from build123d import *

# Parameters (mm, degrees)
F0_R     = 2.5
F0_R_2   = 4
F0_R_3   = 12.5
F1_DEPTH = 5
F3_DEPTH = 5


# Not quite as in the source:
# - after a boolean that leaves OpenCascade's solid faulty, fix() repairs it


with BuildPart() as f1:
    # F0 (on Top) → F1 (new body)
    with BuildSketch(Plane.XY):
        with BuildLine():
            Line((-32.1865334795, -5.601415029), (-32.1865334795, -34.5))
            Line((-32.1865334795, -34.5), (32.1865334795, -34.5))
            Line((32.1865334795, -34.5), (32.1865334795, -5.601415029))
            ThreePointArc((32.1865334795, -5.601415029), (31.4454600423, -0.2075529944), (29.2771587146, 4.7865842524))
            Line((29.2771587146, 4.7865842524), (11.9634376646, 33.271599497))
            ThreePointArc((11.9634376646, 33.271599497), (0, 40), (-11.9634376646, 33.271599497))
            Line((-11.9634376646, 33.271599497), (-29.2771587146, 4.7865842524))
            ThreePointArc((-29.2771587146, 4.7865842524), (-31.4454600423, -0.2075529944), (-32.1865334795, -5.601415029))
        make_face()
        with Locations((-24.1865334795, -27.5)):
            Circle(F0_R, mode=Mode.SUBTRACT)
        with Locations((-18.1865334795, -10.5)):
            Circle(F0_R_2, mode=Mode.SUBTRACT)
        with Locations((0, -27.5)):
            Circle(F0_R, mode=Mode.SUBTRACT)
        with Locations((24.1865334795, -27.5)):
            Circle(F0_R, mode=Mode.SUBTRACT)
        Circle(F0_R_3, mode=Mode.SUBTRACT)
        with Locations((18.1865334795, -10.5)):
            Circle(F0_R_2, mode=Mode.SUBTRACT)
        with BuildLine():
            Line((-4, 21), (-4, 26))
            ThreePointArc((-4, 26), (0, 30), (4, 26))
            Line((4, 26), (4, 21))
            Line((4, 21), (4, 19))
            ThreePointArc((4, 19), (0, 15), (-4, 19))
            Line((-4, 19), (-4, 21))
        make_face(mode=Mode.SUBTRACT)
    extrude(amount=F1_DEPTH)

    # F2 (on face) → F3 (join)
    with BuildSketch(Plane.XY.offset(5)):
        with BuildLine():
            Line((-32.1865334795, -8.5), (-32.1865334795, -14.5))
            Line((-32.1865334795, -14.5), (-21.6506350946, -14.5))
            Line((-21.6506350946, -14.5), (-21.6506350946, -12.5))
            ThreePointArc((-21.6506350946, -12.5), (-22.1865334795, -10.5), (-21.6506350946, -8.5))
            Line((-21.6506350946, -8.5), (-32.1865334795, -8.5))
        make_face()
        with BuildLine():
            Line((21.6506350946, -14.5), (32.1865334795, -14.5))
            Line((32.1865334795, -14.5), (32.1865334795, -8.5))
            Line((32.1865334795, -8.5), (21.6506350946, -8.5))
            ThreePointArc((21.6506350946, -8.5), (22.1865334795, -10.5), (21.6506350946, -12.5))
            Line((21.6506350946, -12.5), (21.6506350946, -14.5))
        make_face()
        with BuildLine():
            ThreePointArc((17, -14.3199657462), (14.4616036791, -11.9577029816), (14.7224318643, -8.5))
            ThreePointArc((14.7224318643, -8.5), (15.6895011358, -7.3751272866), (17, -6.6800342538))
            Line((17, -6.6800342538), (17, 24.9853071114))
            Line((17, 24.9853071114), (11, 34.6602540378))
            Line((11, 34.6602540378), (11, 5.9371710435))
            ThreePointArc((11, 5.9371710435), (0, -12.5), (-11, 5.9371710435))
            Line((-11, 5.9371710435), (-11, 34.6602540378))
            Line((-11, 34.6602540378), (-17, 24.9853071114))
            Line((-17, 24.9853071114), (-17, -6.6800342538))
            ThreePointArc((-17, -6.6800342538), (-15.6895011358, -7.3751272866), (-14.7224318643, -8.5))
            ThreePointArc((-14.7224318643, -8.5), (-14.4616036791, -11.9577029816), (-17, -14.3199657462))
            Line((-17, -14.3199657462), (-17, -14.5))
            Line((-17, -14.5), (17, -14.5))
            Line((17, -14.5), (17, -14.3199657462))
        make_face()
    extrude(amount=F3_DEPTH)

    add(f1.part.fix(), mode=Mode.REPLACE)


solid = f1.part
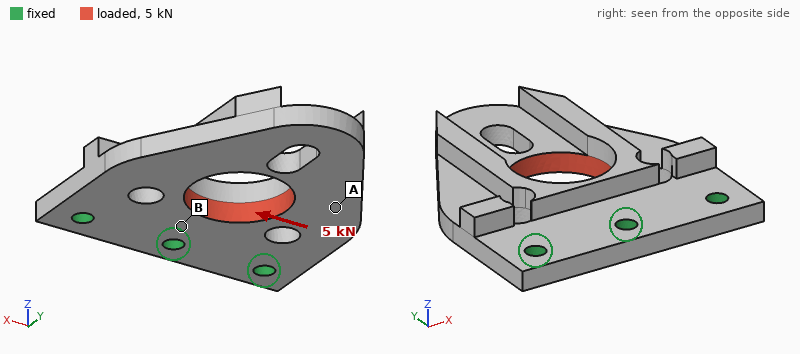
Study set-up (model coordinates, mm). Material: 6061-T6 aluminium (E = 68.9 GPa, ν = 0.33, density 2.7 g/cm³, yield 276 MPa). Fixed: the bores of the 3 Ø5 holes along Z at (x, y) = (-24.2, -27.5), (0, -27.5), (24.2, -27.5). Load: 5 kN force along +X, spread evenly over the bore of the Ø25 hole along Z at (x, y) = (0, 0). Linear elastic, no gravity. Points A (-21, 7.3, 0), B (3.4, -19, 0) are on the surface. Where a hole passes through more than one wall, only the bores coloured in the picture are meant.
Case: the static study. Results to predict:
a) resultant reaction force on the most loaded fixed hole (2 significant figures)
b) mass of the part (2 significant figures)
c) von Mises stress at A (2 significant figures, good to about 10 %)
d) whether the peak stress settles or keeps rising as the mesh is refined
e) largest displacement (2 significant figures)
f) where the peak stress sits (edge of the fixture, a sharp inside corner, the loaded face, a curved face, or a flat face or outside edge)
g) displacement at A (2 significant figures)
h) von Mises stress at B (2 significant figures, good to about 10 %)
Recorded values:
2.8 kN
50 g
21 MPa
keeps rising
67 µm
edge of the fixture
52 µm
51 MPa
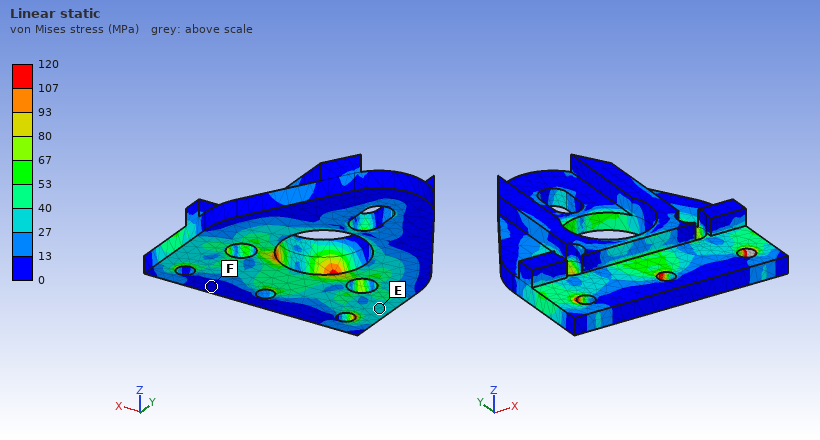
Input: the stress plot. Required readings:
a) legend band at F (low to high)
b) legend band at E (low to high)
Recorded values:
0 to 13 MPa
27 to 40 MPa
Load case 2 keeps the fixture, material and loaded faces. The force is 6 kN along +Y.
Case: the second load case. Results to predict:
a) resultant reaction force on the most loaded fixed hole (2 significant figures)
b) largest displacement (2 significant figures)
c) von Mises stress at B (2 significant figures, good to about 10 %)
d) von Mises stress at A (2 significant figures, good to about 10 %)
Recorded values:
2.1 kN
66 µm
22 MPa
19 MPa
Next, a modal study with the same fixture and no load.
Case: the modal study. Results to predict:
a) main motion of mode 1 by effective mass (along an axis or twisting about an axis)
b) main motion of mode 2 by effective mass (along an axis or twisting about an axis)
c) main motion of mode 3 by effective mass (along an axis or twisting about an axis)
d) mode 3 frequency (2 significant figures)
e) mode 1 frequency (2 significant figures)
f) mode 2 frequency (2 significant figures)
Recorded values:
along Z
twisting about Y
along X
7200 Hz
1300 Hz
3700 Hz
